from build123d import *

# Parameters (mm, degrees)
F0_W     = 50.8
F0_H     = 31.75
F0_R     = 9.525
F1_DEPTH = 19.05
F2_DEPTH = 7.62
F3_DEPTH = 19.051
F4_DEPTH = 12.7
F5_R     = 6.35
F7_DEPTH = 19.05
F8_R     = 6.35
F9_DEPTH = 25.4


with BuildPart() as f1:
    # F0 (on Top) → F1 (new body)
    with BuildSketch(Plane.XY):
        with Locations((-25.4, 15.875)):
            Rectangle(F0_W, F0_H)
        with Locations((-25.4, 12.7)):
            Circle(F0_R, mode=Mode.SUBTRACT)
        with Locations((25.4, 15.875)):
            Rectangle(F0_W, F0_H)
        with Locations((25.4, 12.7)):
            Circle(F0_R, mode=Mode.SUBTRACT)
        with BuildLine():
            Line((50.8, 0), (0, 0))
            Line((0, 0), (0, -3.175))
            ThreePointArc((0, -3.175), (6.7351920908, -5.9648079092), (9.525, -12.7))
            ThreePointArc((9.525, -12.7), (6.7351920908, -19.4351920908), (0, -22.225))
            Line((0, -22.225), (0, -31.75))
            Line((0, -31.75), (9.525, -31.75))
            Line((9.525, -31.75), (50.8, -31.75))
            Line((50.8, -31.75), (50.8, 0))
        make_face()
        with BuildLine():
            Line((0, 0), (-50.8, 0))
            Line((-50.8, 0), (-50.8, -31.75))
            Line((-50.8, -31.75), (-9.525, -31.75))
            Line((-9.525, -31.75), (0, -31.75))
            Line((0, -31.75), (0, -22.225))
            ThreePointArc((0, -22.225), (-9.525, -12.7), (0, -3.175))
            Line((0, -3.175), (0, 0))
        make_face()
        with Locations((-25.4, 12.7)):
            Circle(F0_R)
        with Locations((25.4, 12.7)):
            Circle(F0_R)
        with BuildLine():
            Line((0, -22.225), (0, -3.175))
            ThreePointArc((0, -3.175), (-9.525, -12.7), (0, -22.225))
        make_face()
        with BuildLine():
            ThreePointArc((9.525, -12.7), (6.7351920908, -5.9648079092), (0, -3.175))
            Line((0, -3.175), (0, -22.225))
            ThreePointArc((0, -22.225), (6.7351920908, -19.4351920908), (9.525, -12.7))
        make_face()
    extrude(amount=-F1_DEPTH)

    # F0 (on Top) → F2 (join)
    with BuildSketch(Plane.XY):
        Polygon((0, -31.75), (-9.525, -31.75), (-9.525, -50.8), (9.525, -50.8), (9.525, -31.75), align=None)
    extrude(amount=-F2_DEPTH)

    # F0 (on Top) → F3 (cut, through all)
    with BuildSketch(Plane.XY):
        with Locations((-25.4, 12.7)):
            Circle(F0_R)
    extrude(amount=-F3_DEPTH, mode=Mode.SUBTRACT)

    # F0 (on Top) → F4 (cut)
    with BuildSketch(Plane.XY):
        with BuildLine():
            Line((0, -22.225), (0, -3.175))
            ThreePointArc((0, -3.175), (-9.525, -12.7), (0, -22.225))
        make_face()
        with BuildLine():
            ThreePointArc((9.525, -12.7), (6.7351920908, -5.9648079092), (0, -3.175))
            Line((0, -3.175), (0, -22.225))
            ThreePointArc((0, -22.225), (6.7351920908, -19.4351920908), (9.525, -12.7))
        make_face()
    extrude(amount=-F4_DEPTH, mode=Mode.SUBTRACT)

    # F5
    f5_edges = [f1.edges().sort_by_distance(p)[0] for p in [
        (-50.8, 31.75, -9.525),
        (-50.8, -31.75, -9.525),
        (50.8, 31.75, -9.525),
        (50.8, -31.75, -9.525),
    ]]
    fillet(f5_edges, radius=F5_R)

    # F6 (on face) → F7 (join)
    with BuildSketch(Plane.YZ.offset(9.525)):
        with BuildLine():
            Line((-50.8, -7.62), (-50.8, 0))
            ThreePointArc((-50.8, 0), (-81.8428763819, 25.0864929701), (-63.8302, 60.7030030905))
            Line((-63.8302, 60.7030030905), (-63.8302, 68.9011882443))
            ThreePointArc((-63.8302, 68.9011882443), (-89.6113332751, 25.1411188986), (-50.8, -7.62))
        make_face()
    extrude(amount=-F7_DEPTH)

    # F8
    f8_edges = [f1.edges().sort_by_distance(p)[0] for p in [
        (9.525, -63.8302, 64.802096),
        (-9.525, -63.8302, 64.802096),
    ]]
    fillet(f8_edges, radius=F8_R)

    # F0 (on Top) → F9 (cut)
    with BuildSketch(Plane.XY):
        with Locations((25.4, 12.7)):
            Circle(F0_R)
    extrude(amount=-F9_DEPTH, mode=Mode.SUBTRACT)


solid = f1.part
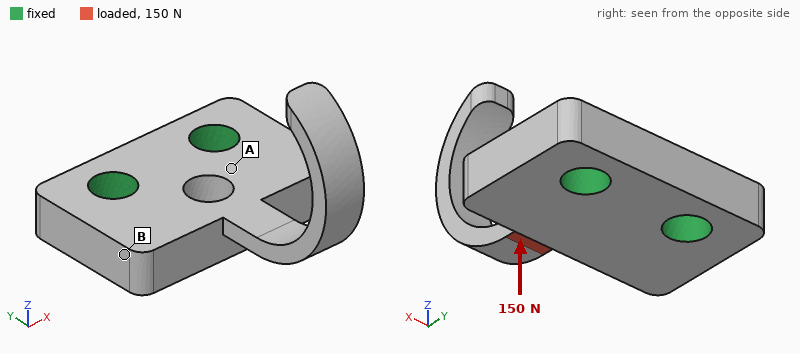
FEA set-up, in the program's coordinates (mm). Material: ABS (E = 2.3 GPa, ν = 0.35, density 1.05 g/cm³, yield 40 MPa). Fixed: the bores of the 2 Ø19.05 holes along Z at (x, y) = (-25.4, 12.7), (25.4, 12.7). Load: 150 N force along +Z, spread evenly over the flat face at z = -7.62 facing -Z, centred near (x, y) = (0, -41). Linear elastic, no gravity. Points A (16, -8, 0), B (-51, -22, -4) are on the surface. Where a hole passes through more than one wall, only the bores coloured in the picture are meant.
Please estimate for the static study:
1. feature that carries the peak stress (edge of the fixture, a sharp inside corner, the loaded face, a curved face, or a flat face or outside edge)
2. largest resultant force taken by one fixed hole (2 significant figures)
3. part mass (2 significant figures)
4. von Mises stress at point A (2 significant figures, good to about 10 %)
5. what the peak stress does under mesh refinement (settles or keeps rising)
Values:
a sharp inside corner
75 N
130 g
1.4 MPa
keeps rising
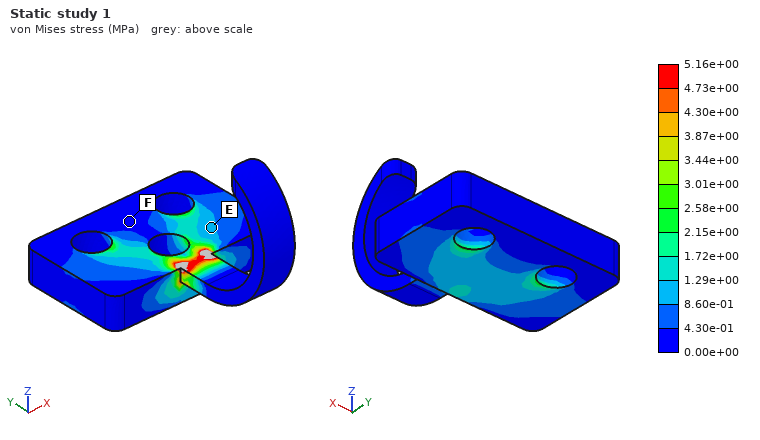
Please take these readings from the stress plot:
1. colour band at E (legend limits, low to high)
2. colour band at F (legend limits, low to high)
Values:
8.60e-01 to 1.29e+00 MPa
0.00e+00 to 4.30e-01 MPa
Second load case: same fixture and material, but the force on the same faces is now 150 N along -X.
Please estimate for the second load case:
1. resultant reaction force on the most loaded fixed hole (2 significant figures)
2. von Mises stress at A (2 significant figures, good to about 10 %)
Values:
140 N
0.44 MPa
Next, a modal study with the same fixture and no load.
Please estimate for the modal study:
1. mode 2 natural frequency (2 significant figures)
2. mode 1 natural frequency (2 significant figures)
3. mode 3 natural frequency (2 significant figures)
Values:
210 Hz
150 Hz
460 Hz
